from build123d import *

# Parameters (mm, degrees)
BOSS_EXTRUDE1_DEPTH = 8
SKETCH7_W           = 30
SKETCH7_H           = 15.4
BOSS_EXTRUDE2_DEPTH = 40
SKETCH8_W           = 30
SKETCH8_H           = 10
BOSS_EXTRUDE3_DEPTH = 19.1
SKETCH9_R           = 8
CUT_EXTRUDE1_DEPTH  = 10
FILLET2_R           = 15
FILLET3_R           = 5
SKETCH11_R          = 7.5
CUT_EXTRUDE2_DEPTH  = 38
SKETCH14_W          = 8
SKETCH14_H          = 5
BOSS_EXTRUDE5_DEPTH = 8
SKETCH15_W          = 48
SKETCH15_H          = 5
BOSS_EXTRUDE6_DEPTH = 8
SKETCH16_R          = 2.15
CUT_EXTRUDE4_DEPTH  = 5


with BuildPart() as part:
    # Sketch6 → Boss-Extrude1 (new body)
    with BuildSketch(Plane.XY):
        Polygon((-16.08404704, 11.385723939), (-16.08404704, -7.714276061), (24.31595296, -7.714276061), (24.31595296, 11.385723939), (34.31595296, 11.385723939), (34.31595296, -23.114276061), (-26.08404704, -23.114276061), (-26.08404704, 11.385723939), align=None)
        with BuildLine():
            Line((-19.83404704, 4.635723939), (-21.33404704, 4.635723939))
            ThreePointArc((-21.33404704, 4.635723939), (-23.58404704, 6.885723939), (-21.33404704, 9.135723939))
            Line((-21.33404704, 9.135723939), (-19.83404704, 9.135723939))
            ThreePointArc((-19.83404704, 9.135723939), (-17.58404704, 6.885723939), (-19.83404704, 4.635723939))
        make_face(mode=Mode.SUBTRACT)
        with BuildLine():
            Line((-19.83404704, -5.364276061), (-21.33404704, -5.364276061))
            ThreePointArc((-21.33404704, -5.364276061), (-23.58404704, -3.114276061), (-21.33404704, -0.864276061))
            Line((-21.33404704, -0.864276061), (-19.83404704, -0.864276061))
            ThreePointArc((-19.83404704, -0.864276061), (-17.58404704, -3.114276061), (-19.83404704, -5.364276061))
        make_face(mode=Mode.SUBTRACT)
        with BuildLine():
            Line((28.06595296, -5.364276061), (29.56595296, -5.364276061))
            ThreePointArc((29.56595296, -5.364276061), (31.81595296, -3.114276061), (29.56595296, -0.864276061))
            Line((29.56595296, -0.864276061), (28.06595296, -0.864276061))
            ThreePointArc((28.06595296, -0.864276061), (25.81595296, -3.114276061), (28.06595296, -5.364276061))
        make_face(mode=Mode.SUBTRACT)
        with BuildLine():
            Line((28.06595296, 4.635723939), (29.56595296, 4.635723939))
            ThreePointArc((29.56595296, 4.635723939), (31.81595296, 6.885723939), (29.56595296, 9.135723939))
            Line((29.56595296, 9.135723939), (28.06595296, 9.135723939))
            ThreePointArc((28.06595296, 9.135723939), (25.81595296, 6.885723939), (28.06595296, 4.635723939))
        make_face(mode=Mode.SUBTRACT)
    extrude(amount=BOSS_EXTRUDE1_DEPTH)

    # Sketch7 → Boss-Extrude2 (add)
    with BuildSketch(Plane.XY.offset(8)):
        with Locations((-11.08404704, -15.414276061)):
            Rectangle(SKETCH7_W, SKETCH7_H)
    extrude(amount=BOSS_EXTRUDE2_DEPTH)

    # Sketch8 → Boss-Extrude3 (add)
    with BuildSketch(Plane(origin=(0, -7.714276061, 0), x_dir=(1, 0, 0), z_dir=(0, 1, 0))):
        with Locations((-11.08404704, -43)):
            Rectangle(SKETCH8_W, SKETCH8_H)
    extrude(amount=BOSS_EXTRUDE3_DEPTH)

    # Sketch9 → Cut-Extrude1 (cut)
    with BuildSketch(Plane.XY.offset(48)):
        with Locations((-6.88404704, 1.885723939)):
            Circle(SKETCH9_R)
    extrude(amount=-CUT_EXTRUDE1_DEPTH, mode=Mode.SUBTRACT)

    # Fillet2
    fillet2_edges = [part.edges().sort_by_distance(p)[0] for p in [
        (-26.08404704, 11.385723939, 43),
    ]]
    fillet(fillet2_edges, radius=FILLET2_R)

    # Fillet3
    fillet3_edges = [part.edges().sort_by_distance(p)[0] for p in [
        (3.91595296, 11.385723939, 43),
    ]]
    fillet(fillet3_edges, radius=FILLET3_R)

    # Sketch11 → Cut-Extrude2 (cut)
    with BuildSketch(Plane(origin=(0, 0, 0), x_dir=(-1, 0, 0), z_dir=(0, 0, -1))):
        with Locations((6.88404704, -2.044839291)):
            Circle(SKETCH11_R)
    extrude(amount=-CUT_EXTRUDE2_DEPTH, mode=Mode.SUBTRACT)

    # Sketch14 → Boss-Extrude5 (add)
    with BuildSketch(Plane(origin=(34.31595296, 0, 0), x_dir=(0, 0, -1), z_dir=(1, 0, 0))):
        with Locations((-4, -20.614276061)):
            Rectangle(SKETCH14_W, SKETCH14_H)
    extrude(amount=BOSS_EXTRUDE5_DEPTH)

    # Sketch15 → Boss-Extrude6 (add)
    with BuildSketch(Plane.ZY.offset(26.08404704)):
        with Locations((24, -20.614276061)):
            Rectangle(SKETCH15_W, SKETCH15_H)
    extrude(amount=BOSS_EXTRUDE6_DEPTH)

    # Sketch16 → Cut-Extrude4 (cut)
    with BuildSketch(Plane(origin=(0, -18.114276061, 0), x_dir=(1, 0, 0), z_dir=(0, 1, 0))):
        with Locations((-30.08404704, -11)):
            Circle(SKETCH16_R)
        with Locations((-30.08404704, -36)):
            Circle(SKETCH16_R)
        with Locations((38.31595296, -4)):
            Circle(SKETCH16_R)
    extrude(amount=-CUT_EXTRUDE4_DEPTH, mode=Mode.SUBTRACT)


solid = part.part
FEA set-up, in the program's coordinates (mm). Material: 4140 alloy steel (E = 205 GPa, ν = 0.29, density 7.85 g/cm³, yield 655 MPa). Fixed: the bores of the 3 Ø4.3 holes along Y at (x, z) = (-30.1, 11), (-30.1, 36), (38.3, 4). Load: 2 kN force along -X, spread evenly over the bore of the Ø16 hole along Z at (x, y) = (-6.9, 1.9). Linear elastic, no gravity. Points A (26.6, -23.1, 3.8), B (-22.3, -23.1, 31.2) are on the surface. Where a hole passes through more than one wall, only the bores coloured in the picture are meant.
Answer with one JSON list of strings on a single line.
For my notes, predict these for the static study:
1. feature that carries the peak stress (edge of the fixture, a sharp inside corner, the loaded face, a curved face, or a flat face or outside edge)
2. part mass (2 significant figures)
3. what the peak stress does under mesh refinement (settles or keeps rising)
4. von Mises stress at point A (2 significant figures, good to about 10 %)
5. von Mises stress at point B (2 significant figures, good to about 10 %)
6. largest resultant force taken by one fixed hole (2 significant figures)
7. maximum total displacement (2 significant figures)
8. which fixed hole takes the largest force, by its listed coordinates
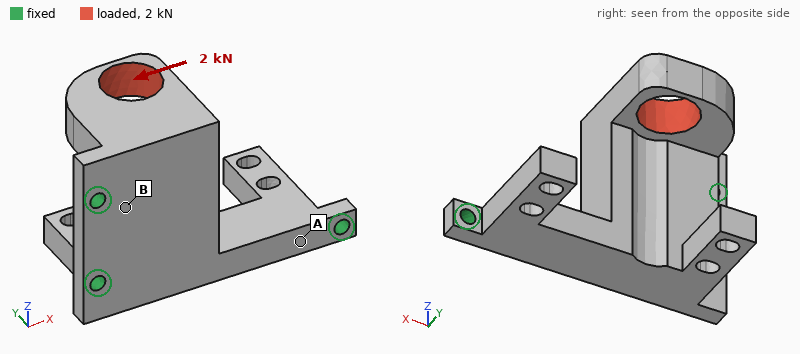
["edge of the fixture", "260 g", "keeps rising", "15 MPa", "39 MPa", "2.2 kN", "56 µm", "(-30.1, 36)"]
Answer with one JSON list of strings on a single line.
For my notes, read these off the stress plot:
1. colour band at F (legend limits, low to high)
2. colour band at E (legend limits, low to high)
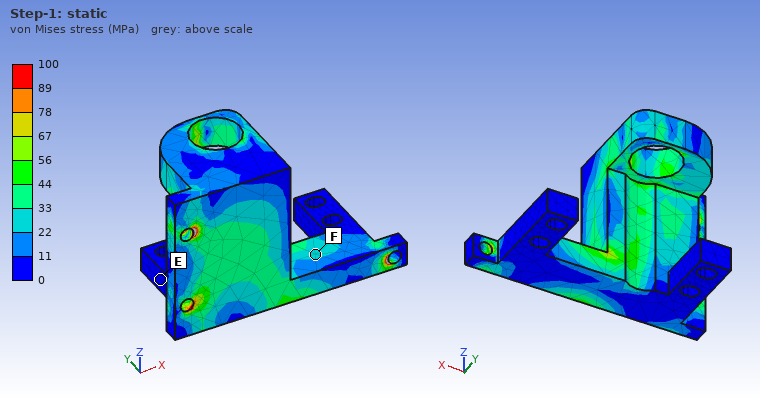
["22 to 33 MPa", "0 to 11 MPa"]
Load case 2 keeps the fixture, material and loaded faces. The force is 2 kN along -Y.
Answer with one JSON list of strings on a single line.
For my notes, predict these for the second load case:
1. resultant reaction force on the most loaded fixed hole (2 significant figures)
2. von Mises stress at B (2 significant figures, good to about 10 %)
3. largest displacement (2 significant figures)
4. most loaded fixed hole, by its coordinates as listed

["2.4 kN", "41 MPa", "54 µm", "(-30.1, 36)"]
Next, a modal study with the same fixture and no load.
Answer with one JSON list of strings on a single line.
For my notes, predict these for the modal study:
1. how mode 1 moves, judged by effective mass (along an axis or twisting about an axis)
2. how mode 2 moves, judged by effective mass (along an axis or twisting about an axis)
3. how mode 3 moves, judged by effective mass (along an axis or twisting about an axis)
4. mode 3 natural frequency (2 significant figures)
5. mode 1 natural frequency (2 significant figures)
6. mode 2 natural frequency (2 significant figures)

["along Y", "along Z", "along Z", "7000 Hz", "4000 Hz", "5500 Hz"]
